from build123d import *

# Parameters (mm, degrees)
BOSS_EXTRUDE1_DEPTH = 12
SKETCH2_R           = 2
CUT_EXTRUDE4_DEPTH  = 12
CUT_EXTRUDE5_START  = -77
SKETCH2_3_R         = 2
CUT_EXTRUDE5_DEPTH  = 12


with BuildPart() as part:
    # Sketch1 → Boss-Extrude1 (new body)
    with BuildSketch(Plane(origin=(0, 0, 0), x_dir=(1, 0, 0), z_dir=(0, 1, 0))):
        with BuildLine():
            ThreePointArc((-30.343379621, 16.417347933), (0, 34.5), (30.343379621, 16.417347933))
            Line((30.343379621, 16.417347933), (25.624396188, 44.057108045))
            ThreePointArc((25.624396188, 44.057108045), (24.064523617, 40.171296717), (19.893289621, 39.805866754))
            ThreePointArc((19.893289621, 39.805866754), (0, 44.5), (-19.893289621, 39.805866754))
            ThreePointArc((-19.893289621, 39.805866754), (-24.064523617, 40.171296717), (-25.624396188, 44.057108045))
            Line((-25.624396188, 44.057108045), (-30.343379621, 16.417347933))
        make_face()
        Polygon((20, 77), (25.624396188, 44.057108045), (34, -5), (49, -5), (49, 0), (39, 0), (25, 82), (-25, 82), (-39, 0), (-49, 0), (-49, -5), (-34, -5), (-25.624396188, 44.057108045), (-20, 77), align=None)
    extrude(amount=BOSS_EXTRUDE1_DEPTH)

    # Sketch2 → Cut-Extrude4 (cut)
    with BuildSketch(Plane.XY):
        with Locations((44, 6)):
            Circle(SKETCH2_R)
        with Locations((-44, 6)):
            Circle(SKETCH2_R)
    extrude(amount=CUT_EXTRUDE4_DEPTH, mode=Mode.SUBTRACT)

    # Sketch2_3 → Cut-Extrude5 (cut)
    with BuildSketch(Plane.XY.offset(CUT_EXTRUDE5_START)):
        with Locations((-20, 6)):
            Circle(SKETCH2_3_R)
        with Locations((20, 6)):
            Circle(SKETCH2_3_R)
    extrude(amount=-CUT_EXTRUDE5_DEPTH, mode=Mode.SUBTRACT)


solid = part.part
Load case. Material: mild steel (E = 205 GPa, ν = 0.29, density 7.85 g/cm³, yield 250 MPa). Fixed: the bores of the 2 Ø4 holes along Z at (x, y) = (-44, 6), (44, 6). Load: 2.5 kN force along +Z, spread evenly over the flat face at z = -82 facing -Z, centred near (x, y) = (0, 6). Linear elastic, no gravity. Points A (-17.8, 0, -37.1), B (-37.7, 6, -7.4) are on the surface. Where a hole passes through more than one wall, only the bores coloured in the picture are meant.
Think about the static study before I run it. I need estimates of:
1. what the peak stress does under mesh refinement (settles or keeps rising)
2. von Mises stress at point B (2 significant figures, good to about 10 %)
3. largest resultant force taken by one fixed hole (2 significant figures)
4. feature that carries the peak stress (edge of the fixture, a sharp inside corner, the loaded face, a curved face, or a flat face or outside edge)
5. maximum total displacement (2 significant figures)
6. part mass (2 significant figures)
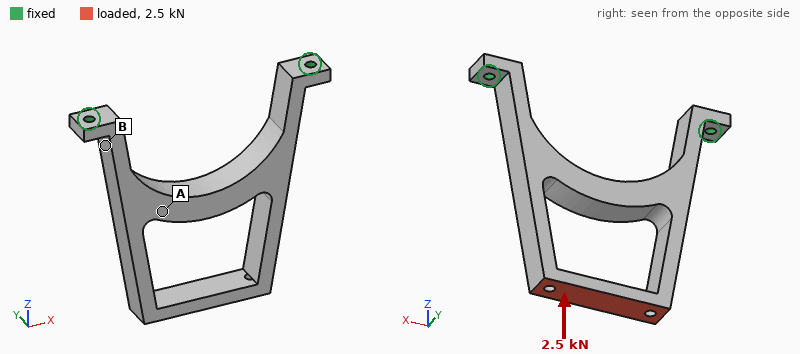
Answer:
keeps rising
43 MPa
1.3 kN
a sharp inside corner
59 µm
190 g
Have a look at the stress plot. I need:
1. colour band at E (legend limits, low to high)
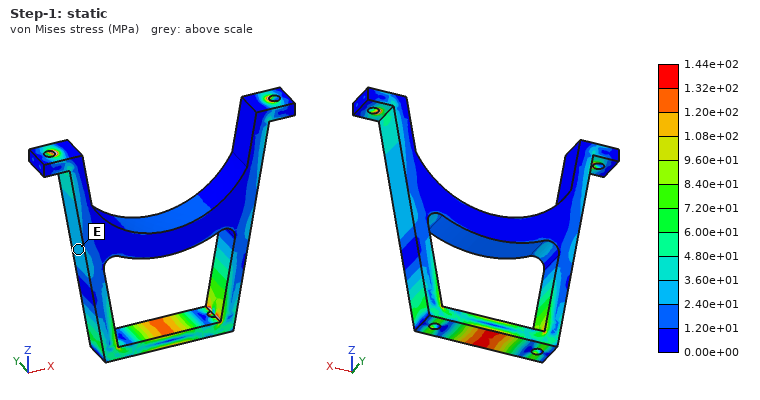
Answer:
2.40e+01 to 3.60e+01 MPa
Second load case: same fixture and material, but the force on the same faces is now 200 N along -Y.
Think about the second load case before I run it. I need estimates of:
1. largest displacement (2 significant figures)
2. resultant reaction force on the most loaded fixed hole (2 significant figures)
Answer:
0.23 mm
100 N
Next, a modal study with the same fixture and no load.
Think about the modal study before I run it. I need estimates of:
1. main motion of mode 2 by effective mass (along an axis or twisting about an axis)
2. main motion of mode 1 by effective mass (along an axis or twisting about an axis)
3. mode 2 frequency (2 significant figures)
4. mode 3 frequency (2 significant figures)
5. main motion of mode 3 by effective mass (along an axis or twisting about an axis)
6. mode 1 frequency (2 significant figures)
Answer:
along X
along Y
2000 Hz
2100 Hz
twisting about Z
650 Hz
